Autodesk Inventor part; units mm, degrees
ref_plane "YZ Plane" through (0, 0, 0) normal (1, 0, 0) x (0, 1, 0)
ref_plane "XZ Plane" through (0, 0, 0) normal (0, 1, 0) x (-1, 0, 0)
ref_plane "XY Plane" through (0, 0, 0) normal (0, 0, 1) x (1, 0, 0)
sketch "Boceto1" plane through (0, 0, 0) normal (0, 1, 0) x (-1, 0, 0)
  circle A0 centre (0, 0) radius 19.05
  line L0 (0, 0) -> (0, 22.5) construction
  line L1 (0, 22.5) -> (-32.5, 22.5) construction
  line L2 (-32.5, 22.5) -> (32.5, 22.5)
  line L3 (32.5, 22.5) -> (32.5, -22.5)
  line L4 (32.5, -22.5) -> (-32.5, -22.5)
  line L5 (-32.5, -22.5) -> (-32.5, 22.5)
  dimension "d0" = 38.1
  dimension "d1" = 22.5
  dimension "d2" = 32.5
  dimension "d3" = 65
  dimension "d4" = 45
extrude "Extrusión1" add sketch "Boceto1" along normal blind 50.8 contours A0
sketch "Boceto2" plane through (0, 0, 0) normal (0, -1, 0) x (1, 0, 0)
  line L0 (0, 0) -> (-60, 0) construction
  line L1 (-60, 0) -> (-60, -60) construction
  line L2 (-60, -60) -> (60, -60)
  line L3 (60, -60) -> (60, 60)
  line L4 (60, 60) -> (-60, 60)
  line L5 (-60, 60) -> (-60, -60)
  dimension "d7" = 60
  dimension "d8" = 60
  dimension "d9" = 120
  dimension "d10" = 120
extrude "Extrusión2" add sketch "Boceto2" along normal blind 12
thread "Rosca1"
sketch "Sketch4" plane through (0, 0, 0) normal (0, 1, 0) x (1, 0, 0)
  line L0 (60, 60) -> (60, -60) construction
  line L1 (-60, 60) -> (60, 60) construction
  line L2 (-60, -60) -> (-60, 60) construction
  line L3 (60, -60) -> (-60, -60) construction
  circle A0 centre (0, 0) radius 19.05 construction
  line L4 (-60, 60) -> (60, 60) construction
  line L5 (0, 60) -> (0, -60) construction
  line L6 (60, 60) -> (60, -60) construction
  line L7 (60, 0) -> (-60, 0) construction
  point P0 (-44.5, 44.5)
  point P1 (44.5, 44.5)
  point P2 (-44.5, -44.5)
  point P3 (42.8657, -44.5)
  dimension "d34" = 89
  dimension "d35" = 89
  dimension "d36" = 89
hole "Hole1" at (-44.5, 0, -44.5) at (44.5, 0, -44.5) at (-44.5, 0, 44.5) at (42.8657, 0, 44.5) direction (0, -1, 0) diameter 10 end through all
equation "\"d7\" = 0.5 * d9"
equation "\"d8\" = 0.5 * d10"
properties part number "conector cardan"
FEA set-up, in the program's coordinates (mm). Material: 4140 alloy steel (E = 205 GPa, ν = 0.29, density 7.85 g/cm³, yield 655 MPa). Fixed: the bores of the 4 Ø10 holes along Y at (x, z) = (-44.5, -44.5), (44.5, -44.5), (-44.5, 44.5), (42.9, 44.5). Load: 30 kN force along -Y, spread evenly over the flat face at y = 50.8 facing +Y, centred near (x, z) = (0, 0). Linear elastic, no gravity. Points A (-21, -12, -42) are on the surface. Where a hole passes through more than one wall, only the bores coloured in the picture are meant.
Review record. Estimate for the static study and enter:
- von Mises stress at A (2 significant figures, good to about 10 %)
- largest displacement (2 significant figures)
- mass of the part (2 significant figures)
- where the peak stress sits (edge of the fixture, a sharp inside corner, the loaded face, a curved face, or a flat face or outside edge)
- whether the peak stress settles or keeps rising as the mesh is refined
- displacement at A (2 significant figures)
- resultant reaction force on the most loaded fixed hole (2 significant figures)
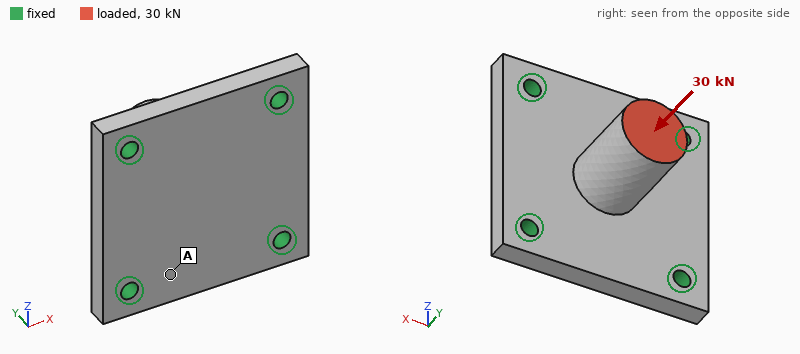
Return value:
46 MPa
68 µm
1.8 kg
edge of the fixture
keeps rising
20 µm
7.8 kN
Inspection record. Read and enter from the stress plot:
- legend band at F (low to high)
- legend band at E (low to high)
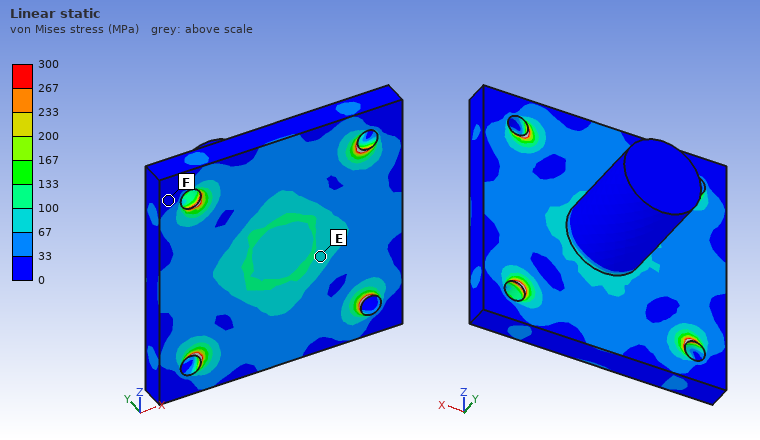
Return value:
0 to 33 MPa
67 to 100 MPa
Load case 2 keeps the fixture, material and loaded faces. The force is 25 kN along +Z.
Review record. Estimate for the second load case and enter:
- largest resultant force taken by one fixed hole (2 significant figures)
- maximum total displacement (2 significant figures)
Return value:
12 kN
0.25 mm
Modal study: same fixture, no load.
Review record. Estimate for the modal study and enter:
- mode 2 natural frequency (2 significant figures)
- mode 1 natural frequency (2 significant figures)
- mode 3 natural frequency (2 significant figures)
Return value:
3800 Hz
3800 Hz
3900 Hz
